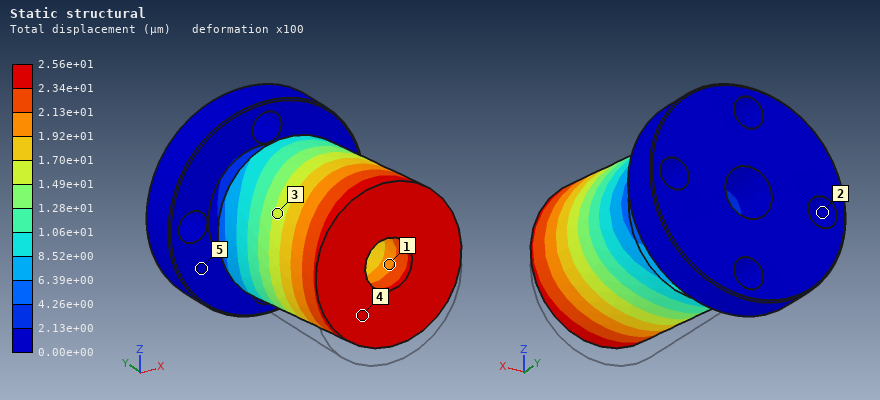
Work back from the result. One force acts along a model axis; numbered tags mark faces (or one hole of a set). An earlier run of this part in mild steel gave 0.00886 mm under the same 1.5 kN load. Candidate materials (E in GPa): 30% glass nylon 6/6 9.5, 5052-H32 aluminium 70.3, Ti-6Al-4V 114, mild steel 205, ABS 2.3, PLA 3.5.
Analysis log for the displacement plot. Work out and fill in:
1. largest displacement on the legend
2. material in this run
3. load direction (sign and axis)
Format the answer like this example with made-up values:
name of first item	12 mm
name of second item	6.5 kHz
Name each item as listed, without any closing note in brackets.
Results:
largest displacement on the legend	2.56e+01 µm
material in this run	5052-H32 aluminium
load direction	+Z
